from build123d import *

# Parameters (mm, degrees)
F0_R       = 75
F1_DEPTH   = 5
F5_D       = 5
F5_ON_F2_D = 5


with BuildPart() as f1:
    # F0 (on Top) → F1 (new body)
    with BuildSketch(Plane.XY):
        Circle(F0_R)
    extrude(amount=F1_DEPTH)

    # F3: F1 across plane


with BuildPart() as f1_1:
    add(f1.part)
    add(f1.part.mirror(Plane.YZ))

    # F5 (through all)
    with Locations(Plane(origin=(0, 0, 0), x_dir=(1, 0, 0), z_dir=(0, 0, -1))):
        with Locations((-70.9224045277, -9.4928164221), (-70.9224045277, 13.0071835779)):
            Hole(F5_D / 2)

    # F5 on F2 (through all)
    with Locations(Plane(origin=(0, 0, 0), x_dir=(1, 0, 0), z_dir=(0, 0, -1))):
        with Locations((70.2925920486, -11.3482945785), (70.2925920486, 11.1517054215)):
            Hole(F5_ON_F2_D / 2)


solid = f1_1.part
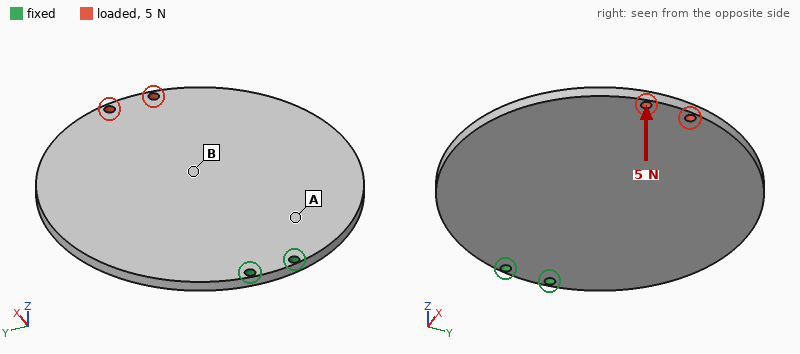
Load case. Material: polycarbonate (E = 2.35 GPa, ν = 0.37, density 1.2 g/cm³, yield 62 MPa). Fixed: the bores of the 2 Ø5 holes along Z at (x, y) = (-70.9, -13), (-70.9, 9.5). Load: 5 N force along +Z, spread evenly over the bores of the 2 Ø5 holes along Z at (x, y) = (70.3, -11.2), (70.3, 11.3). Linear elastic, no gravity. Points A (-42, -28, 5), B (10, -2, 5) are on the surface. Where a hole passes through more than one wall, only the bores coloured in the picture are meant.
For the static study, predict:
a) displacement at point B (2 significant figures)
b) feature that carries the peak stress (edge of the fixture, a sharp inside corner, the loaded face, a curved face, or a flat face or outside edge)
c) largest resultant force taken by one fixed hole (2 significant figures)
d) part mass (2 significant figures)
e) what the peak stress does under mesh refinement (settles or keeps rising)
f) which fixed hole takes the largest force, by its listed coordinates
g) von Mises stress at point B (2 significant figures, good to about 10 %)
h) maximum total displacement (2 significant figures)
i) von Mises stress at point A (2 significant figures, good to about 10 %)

1.0 mm
edge of the fixture
3.0 N
110 g
keeps rising
(-70.9, 9.5)
0.51 MPa
2.3 mm
1.2 MPa
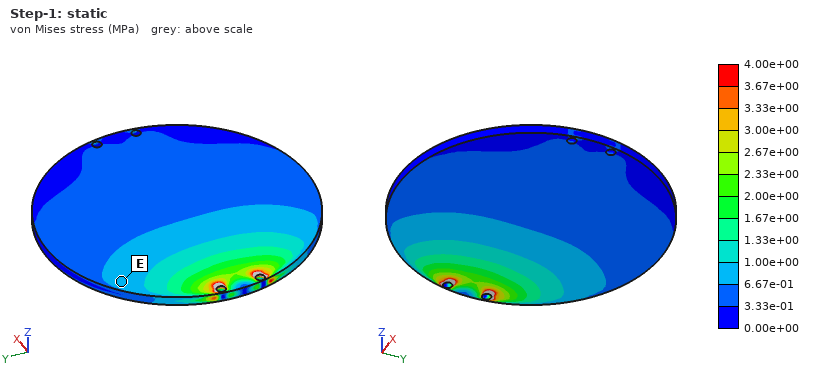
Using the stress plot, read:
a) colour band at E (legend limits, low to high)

6.67e-01 to 1.00e+00 MPa
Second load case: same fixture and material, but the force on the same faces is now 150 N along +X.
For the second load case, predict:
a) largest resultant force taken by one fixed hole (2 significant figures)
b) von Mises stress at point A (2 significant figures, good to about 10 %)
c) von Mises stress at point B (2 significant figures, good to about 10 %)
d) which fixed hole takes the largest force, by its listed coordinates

86 N
0.32 MPa
0.44 MPa
(-70.9, 9.5)
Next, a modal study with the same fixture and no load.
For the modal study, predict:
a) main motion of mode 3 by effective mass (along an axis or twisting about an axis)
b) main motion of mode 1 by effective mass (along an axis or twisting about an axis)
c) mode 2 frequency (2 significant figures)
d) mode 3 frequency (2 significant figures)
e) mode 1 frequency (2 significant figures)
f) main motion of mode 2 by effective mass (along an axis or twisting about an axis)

along Z
along Z
100 Hz
260 Hz
47 Hz
twisting about X
